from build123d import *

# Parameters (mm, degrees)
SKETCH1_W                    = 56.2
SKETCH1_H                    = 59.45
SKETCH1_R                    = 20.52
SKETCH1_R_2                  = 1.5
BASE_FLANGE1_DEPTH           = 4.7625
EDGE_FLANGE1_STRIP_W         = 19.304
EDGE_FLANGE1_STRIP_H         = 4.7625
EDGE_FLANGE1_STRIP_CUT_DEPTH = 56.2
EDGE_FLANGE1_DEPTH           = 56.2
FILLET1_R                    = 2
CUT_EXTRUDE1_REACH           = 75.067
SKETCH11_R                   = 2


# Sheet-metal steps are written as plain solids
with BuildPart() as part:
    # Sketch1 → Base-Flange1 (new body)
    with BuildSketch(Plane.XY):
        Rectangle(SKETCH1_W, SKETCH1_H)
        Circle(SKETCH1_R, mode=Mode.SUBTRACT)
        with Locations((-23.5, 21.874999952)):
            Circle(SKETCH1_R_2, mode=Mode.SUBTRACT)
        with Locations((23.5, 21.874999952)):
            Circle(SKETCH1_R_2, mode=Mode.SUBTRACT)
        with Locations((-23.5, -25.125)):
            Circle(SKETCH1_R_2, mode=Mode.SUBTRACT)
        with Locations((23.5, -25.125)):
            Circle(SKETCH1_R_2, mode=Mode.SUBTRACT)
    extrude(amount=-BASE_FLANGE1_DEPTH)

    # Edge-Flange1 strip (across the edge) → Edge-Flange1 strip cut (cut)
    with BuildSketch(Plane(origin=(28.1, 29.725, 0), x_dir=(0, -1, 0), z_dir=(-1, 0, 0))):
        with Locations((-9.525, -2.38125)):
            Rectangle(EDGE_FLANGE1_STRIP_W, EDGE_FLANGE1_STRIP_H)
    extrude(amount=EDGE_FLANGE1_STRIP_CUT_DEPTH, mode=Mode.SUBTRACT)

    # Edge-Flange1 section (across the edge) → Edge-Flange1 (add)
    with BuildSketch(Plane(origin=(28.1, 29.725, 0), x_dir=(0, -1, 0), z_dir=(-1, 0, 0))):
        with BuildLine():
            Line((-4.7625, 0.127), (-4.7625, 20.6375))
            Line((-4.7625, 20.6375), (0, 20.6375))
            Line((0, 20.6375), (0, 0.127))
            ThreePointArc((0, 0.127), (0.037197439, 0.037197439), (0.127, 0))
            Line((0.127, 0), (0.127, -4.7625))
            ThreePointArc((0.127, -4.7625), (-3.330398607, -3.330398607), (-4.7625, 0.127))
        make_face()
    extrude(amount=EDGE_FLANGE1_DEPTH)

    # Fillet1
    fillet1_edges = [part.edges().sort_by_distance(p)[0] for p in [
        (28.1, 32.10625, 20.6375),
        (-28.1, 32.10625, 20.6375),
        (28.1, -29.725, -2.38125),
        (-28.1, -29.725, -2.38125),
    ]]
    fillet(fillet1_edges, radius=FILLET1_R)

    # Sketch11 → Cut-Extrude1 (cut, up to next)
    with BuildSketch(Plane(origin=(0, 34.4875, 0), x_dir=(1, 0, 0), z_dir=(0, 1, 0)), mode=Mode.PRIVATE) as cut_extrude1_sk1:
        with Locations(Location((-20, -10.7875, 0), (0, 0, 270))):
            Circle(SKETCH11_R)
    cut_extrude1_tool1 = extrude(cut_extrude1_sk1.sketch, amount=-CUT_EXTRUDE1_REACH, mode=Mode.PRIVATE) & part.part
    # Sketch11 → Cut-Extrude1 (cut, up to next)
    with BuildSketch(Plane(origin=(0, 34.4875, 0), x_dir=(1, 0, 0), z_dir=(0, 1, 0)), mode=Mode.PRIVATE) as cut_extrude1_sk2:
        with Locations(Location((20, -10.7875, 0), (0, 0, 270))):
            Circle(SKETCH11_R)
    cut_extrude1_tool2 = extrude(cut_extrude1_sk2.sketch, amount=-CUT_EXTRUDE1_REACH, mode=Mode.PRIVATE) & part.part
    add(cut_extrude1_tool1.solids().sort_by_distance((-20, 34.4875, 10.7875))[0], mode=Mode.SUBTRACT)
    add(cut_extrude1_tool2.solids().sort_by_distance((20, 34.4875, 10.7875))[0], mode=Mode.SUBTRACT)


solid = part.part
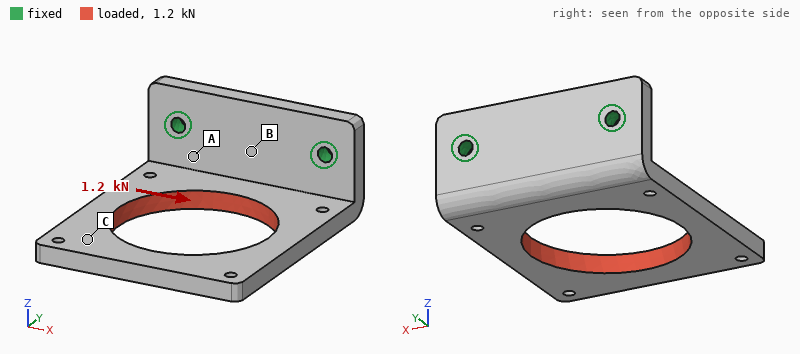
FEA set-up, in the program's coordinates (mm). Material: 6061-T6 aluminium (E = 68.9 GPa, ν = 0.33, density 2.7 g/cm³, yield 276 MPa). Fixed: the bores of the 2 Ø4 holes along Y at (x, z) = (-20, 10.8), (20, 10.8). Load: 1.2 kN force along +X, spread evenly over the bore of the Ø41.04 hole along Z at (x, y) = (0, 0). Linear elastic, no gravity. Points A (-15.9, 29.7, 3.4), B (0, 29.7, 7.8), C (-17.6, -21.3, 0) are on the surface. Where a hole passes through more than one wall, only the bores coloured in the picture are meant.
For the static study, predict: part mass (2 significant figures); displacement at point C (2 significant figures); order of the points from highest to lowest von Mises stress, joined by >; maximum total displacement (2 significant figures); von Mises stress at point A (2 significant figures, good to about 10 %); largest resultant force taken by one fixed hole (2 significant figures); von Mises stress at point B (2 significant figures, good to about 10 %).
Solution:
43 g
0.20 mm
A > B > C
0.23 mm
55 MPa
1.1 kN
24 MPa
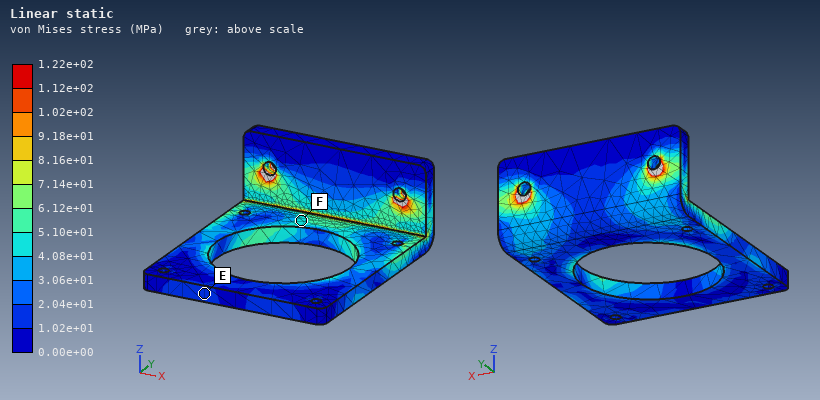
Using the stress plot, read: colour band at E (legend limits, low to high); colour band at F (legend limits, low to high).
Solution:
1.02e+01 to 2.04e+01 MPa
4.08e+01 to 5.10e+01 MPa
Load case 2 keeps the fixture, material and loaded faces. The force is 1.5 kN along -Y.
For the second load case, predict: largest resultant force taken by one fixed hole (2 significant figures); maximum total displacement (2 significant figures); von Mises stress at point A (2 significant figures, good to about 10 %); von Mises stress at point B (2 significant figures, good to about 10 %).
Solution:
750 N
0.30 mm
43 MPa
21 MPa
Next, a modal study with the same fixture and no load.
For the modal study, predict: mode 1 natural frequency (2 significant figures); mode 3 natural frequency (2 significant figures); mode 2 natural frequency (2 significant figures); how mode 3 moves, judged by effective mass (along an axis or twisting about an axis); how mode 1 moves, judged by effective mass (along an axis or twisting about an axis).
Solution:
710 Hz
2800 Hz
1800 Hz
along X
along Z
